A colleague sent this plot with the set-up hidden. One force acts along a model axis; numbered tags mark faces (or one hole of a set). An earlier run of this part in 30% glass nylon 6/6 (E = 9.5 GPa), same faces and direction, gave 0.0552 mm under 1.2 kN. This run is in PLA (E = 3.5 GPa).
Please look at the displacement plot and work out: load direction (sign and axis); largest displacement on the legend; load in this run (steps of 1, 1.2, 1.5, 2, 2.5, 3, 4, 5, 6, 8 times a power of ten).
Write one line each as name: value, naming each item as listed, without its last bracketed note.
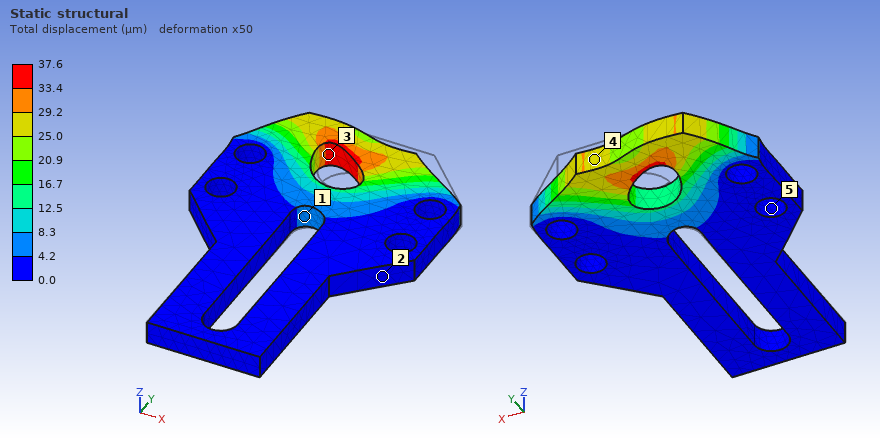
load direction: -X
largest displacement on the legend: 37.6 µm
load in this run: 300 N
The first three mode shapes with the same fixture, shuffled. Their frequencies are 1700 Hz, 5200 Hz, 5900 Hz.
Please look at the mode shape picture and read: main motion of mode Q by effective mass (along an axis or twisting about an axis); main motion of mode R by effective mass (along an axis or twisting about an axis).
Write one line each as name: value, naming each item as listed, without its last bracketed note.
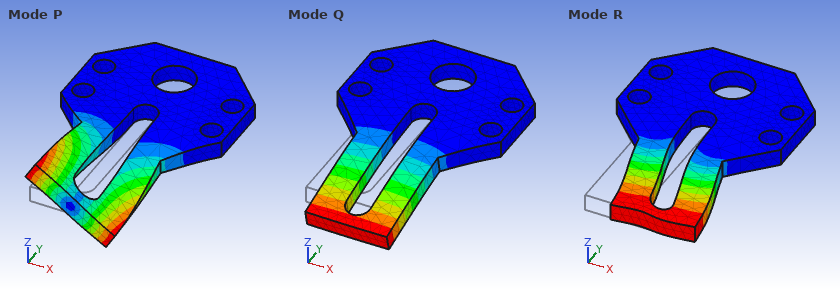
main motion of mode Q by effective mass: along Z
main motion of mode R by effective mass: along X
